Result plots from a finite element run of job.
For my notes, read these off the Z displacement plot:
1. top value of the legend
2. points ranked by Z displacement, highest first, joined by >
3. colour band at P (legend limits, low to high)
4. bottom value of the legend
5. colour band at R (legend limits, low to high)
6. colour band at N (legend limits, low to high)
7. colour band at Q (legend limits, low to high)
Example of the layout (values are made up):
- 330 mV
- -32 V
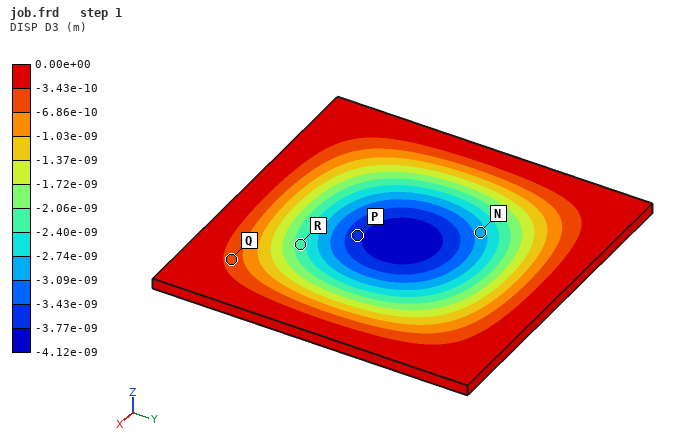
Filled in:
- 0.00e+00 m
- Q > R > N > P
- -3.77e-09 to -3.43e-09 m
- -4.12e-09 m
- -2.40e-09 to -2.06e-09 m
- -3.09e-09 to -2.74e-09 m
- -6.86e-10 to -3.43e-10 m
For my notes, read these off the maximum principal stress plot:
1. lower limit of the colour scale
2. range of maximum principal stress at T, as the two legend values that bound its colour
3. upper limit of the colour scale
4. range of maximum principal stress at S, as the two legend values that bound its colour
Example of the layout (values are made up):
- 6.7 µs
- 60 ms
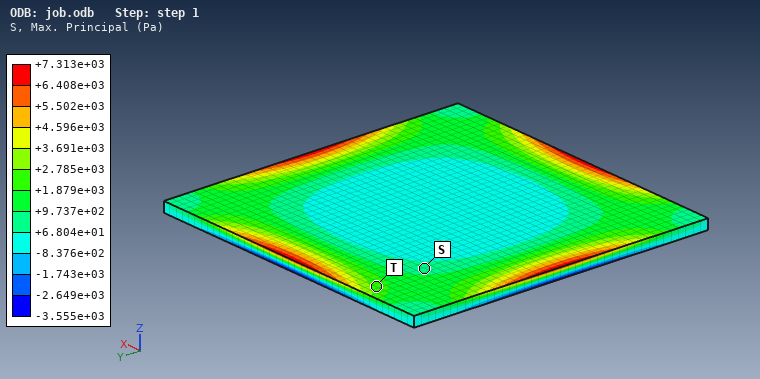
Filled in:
- -3.555e+03 Pa
- +1.879e+03 to +2.785e+03 Pa
- +7.313e+03 Pa
- +6.804e+01 to +9.737e+02 Pa
